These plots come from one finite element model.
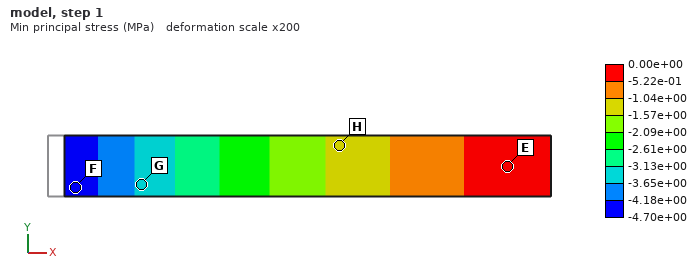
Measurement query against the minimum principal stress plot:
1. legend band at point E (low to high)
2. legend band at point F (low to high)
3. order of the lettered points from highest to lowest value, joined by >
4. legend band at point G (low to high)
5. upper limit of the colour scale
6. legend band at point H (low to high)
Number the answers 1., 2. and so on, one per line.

1. -5.22e-01 to 0.00e+00 MPa
2. -4.70e+00 to -4.18e+00 MPa
3. E > H > G > F
4. -3.65e+00 to -3.13e+00 MPa
5. 0.00e+00 MPa
6. -1.57e+00 to -1.04e+00 MPa
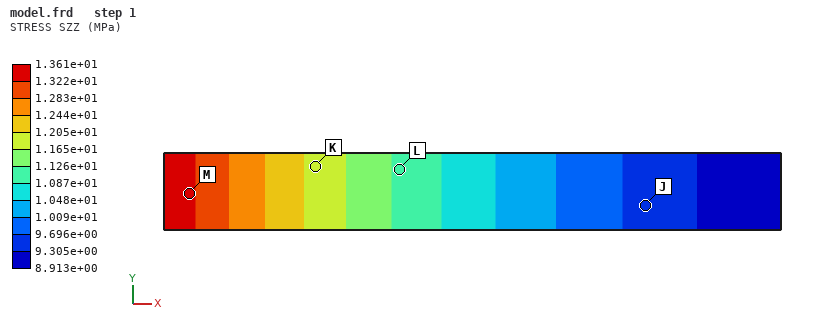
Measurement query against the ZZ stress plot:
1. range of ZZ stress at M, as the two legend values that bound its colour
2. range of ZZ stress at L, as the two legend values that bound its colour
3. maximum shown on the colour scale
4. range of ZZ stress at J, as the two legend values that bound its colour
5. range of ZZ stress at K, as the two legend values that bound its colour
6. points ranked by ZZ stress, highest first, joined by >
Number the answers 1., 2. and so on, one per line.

1. 1.322e+01 to 1.361e+01 MPa
2. 1.087e+01 to 1.126e+01 MPa
3. 1.361e+01 MPa
4. 9.305e+00 to 9.696e+00 MPa
5. 1.165e+01 to 1.205e+01 MPa
6. M > K > L > J
